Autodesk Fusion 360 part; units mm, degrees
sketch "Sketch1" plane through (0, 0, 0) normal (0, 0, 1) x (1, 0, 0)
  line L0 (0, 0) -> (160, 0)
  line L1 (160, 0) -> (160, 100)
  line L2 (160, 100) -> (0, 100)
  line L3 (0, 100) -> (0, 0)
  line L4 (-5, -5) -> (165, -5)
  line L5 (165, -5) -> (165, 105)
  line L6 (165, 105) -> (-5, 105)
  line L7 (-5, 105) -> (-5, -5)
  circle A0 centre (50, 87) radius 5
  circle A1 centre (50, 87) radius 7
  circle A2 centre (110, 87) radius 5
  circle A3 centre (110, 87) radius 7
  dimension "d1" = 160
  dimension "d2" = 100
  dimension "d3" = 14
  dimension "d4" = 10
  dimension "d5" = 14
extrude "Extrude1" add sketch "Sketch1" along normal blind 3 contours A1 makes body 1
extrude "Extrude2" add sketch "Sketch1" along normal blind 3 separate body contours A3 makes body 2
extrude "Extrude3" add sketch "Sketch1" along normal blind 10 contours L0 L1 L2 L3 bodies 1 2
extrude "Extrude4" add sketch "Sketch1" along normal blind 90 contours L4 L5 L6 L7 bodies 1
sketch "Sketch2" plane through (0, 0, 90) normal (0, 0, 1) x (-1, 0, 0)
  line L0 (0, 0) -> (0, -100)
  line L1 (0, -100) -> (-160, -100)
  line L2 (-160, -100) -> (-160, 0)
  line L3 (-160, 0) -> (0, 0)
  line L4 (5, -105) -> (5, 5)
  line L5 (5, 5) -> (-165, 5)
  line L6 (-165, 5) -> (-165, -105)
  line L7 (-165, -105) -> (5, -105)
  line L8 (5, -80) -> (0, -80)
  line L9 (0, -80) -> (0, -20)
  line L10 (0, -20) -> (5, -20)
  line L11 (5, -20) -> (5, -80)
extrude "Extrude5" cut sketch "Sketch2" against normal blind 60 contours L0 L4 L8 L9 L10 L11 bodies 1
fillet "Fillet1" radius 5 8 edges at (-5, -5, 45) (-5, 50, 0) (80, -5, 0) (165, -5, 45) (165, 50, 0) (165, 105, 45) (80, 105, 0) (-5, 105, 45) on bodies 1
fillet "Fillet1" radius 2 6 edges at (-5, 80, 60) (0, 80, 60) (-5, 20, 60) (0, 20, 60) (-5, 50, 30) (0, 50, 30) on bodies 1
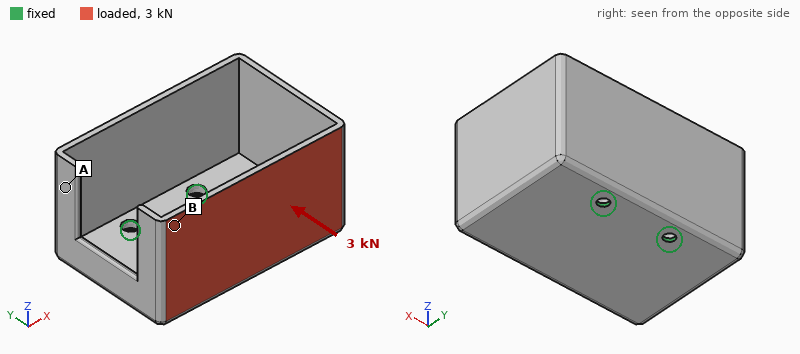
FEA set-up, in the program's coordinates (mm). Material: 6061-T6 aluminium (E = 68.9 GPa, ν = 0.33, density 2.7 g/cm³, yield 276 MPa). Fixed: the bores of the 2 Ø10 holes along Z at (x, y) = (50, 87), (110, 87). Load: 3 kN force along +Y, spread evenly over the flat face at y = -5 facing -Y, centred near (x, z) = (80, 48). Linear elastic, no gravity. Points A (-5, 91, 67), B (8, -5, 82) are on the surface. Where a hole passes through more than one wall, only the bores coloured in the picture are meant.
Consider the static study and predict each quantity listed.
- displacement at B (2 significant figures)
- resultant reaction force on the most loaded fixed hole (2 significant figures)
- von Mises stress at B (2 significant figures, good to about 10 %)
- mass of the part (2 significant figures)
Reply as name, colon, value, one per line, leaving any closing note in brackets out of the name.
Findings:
displacement at B: 1.3 mm
resultant reaction force on the most loaded fixed hole: 1.5 kN
von Mises stress at B: 31 MPa
mass of the part: 1.0 kg
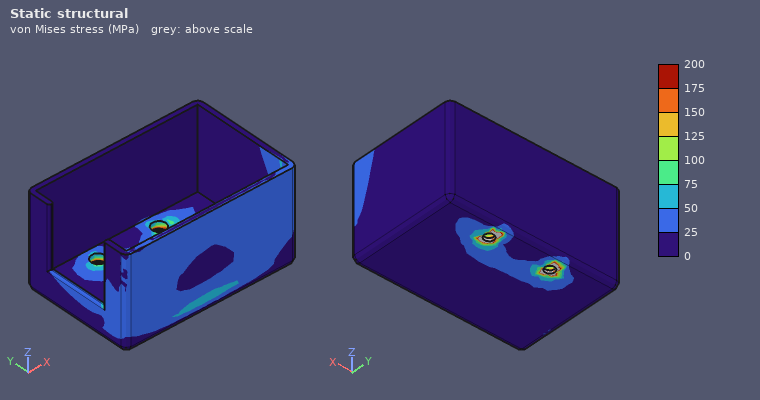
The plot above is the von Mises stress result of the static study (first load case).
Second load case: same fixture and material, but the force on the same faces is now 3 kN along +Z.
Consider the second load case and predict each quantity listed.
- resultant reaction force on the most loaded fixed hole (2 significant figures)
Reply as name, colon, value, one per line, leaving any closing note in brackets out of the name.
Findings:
resultant reaction force on the most loaded fixed hole: 1.8 kN
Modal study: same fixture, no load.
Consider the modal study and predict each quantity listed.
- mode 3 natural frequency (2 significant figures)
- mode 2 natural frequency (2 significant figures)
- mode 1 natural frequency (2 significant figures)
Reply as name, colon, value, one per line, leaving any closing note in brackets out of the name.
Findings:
mode 3 natural frequency: 990 Hz
mode 2 natural frequency: 540 Hz
mode 1 natural frequency: 290 Hz
